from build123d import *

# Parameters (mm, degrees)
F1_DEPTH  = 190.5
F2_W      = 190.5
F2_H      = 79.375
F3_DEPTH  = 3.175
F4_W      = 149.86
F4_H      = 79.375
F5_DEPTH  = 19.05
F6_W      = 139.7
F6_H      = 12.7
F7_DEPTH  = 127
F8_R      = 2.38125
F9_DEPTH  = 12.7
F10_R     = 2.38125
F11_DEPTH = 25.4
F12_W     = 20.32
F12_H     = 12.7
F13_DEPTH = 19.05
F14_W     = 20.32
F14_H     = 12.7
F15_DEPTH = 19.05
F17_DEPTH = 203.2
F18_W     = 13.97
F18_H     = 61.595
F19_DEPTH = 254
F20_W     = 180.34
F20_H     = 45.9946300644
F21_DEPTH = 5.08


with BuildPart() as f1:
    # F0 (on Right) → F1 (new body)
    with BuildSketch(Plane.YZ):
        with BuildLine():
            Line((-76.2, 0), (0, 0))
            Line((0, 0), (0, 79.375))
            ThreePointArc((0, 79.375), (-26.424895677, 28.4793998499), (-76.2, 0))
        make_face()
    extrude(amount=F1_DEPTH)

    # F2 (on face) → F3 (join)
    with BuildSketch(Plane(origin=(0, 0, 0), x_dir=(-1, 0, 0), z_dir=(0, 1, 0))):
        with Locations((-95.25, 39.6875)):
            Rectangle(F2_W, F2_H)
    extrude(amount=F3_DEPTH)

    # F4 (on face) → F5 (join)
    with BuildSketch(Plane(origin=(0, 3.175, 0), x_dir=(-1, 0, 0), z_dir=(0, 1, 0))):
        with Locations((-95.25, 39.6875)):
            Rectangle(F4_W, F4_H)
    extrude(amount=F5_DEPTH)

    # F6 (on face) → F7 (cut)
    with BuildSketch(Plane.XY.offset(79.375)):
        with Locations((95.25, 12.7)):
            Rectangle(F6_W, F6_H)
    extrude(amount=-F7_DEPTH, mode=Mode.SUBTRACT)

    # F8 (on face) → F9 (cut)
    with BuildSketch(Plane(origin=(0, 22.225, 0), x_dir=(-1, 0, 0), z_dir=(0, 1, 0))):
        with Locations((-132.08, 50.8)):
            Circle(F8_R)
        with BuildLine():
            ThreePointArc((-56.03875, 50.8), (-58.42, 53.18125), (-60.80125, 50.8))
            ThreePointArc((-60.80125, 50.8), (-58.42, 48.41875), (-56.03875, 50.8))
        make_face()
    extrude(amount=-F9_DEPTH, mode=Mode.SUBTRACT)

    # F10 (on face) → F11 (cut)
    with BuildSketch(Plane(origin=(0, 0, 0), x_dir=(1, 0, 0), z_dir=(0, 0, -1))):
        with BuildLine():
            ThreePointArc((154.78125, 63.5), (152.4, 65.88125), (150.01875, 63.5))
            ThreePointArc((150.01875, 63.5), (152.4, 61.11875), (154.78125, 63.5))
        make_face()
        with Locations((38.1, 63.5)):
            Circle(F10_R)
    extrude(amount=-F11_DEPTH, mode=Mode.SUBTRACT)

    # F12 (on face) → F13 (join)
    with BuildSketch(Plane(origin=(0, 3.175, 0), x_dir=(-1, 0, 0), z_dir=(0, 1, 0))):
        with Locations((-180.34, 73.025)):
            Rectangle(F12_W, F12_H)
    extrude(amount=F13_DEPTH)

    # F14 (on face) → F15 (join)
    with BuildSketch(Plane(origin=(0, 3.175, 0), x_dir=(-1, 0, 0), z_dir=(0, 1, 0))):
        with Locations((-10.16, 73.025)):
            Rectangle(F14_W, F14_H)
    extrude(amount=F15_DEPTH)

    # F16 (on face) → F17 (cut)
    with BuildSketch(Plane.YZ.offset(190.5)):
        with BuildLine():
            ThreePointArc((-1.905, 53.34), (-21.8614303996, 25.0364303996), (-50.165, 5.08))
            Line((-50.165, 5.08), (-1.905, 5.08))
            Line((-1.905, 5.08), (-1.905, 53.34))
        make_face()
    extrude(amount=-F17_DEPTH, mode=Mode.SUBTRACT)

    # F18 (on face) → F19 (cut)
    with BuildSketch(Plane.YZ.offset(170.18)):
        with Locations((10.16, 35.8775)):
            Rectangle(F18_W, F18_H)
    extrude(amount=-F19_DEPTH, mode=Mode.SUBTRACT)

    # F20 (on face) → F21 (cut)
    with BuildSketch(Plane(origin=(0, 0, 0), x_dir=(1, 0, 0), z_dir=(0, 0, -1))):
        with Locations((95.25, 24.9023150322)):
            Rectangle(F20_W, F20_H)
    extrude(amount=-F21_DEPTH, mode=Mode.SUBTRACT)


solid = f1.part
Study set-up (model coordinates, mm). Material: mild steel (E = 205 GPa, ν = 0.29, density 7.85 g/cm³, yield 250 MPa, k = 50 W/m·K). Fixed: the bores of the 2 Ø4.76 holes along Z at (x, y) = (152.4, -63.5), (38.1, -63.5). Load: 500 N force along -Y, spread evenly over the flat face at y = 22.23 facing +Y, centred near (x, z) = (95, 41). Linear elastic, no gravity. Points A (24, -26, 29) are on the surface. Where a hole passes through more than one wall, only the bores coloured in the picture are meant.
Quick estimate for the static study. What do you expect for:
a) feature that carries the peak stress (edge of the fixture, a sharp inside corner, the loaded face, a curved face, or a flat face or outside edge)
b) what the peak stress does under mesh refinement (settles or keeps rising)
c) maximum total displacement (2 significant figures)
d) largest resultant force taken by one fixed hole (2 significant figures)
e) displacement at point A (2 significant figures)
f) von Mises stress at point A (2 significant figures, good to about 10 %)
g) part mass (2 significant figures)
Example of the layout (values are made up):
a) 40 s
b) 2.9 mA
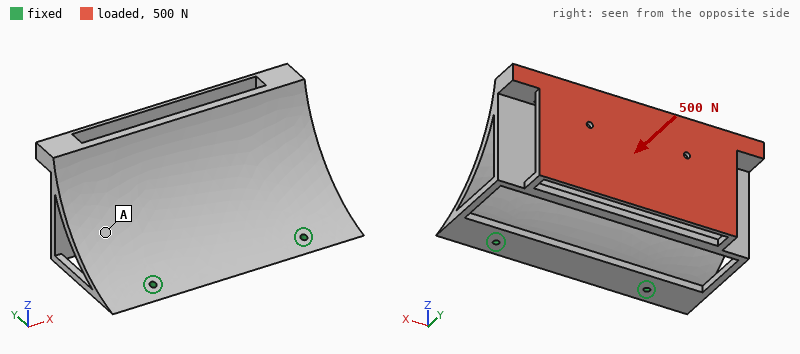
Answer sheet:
a) edge of the fixture
b) keeps rising
c) 0.38 mm
d) 250 N
e) 0.093 mm
f) 8.3 MPa
g) 1.9 kg
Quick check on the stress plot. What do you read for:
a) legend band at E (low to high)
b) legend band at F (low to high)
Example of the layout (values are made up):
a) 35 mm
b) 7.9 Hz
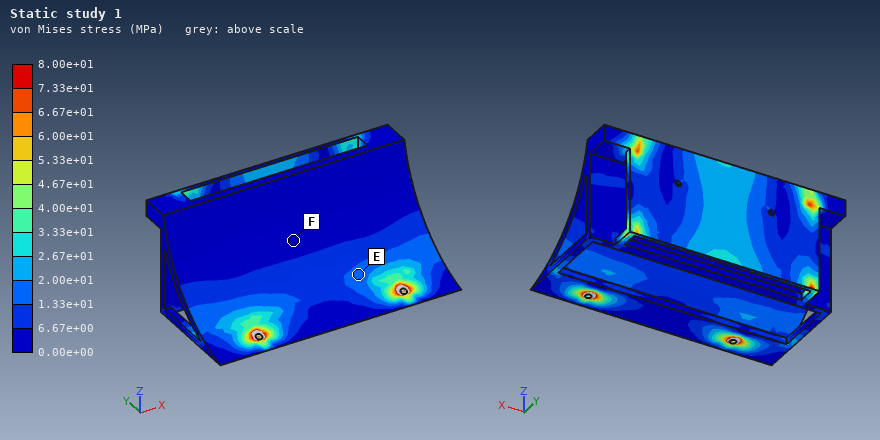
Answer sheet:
a) 1.33e+01 to 2.00e+01 MPa
b) 0.00e+00 to 6.67e+00 MPa
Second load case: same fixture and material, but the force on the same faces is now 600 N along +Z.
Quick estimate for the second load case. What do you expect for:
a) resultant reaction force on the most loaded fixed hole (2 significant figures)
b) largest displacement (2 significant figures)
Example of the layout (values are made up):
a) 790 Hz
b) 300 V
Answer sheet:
a) 430 N
b) 0.75 mm
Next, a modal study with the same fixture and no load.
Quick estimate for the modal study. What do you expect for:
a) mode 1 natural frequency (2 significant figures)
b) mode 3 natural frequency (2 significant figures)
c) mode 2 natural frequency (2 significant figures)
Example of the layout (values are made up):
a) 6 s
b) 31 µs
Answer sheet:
a) 150 Hz
b) 670 Hz
c) 460 Hz
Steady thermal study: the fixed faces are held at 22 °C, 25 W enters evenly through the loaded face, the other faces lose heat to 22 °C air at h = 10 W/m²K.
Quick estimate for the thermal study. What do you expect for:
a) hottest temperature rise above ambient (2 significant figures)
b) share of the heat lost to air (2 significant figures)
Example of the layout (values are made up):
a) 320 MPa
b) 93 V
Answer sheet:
a) 72 K
b) 76 %
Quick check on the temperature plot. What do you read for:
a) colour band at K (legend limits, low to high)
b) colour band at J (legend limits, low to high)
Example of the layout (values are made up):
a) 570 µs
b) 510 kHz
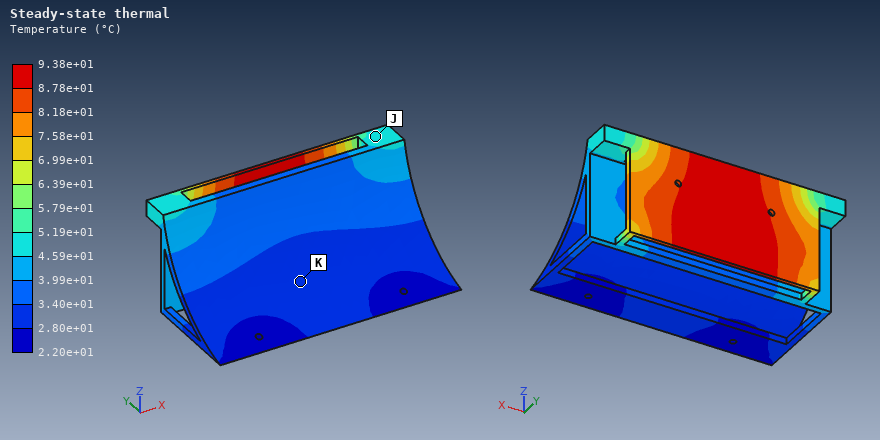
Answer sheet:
a) 2.80e+01 to 3.40e+01 °C
b) 4.59e+01 to 5.19e+01 °C
